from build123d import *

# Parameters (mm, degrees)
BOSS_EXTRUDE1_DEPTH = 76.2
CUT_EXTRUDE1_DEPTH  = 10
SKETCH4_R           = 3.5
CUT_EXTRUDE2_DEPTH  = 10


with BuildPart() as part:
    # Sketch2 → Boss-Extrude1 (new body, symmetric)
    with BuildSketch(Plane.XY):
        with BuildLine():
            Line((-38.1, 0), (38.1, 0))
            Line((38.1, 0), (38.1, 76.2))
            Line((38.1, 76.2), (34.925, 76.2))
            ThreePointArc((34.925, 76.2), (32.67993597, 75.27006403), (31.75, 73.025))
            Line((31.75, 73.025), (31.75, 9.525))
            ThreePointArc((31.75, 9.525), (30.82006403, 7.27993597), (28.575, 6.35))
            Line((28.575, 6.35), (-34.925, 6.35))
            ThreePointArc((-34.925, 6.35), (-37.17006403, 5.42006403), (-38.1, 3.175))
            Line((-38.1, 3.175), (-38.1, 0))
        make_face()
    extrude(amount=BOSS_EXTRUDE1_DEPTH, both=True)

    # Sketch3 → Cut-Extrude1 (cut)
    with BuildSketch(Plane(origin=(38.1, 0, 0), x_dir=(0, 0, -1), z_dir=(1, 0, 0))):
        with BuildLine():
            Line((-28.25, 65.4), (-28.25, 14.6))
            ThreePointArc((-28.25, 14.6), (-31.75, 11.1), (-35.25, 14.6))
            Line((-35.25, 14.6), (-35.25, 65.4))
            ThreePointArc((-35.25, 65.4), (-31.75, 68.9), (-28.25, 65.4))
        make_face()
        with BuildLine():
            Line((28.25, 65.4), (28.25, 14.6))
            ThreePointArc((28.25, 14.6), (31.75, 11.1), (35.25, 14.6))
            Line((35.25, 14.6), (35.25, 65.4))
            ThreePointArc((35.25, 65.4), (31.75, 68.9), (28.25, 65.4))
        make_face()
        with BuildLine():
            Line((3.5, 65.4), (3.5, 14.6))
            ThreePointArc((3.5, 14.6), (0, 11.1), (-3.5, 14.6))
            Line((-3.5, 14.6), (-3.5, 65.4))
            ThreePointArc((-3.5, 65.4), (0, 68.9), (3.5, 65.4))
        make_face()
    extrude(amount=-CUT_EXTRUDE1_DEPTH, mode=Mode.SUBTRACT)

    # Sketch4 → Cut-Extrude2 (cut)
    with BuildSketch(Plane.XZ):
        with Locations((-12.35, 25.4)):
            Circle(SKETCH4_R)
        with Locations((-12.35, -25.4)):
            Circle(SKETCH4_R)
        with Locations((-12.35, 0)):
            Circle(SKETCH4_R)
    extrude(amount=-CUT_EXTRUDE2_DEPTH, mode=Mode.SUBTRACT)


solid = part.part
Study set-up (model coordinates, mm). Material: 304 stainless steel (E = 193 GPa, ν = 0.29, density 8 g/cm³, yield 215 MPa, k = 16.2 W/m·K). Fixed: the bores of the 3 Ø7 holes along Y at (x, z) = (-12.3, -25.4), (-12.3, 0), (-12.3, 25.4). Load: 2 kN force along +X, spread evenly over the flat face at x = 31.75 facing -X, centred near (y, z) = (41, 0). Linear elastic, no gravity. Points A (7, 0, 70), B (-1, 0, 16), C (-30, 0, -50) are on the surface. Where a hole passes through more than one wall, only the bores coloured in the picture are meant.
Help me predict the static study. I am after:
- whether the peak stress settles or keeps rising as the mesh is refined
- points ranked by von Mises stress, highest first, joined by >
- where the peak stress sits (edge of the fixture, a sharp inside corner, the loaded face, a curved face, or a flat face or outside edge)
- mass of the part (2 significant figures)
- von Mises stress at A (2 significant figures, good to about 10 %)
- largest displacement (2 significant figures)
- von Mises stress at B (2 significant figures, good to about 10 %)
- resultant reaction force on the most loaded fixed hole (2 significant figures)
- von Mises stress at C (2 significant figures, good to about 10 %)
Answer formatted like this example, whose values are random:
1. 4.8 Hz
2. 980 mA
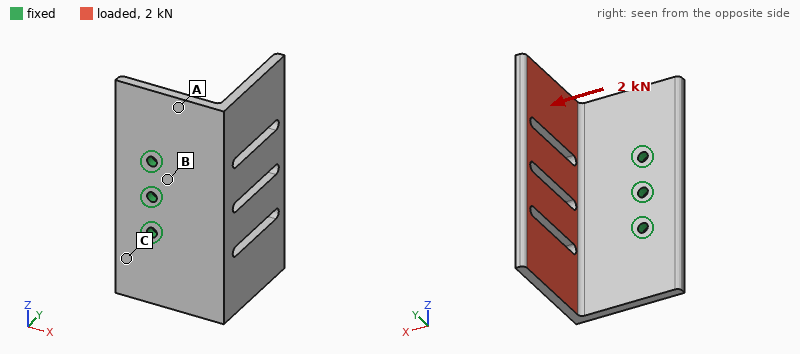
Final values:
1. keeps rising
2. B > A > C
3. edge of the fixture
4. 1.1 kg
5. 59 MPa
6. 0.62 mm
7. 85 MPa
8. 870 N
9. 18 MPa
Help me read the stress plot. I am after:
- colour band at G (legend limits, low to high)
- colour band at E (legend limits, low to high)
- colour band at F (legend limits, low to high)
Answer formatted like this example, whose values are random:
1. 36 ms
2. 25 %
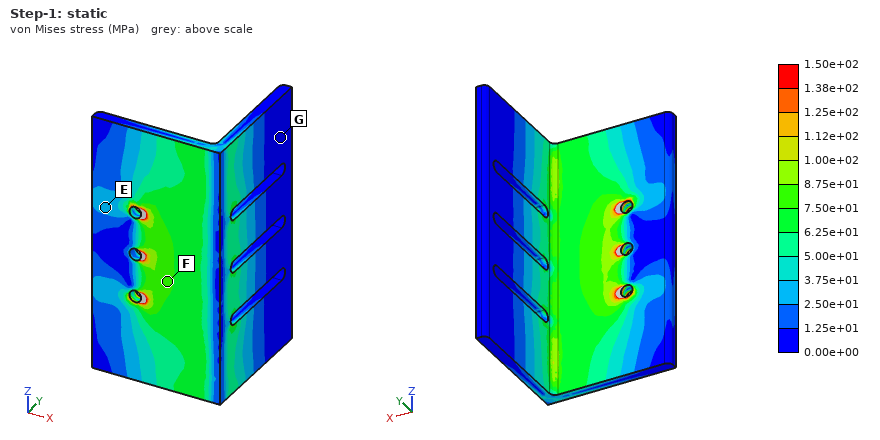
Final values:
1. 0.00e+00 to 1.25e+01 MPa
2. 2.50e+01 to 3.75e+01 MPa
3. 7.50e+01 to 8.75e+01 MPa
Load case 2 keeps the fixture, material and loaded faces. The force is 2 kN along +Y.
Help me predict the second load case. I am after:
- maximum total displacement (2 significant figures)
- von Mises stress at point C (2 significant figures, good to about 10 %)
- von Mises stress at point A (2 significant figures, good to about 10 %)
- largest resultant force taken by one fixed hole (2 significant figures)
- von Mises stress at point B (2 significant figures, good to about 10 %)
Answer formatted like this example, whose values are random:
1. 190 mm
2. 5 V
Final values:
1. 0.28 mm
2. 19 MPa
3. 27 MPa
4. 740 N
5. 83 MPa
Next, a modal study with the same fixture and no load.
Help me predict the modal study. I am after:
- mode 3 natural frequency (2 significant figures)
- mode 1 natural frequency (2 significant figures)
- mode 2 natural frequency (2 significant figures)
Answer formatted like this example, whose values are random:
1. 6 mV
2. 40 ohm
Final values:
1. 1200 Hz
2. 460 Hz
3. 630 Hz
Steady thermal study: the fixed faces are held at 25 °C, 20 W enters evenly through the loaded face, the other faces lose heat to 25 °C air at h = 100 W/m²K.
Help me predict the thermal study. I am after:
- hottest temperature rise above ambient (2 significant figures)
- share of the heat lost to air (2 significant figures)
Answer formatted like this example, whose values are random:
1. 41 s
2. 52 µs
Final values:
1. 14 K
2. 97 %
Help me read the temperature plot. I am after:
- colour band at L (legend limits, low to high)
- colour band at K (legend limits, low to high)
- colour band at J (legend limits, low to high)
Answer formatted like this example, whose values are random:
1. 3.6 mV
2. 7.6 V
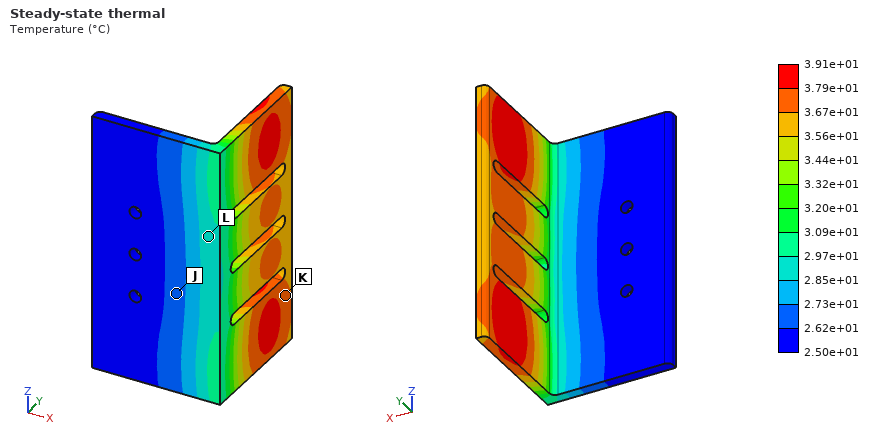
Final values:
1. 2.85e+01 to 2.97e+01 °C
2. 3.67e+01 to 3.79e+01 °C
3. 2.62e+01 to 2.73e+01 °C
